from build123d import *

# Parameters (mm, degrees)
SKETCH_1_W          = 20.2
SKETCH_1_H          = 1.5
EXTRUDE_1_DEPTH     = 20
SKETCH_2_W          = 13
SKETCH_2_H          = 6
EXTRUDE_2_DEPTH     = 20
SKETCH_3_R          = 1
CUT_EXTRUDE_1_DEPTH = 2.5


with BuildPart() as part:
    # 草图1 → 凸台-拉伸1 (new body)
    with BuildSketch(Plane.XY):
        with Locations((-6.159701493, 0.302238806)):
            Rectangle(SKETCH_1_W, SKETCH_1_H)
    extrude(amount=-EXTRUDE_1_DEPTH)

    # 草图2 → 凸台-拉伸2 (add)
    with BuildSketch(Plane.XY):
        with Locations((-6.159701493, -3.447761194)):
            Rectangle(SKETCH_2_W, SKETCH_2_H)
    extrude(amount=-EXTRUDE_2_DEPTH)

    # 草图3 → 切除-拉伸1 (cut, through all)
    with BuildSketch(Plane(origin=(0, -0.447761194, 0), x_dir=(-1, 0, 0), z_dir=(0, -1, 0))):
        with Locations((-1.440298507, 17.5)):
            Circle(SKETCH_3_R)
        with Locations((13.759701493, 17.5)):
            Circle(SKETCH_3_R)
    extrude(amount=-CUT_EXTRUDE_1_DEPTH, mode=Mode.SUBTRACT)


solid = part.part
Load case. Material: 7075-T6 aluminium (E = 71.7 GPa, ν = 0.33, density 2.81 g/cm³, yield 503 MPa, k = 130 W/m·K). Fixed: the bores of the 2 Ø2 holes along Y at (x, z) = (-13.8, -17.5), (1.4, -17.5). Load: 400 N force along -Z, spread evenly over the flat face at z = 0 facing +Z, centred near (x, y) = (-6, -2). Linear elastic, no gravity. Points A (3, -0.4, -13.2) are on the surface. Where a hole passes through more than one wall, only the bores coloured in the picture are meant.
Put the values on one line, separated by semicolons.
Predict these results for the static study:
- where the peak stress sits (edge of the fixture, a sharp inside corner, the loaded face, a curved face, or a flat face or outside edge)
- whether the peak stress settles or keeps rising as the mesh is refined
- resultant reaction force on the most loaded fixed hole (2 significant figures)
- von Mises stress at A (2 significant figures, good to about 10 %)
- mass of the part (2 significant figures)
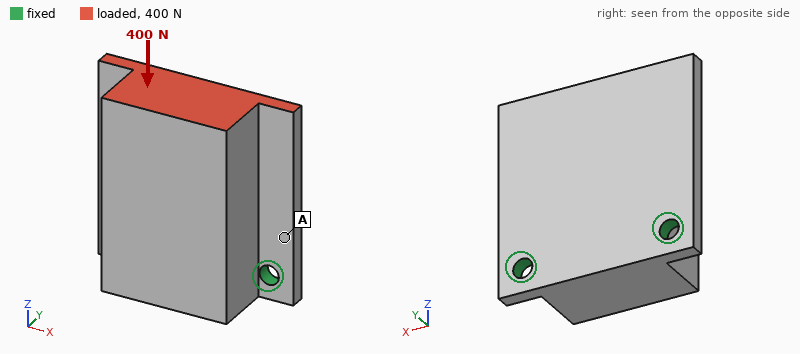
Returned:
edge of the fixture; keeps rising; 200 N; 22 MPa; 6.1 g
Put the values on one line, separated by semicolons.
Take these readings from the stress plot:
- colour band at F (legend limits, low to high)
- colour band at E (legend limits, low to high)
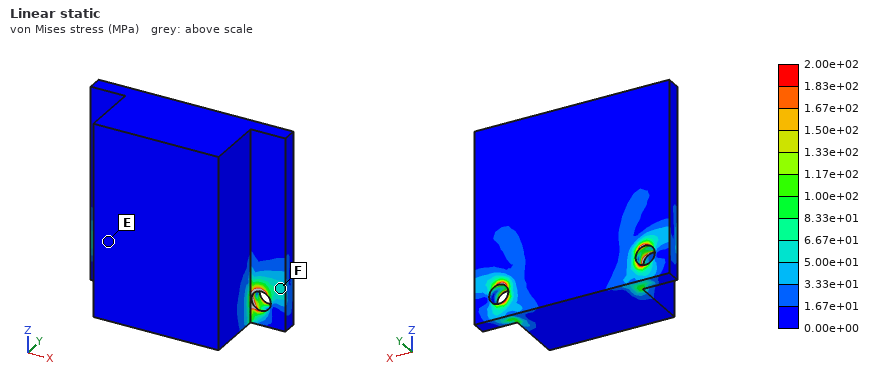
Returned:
5.00e+01 to 6.67e+01 MPa; 0.00e+00 to 1.67e+01 MPa
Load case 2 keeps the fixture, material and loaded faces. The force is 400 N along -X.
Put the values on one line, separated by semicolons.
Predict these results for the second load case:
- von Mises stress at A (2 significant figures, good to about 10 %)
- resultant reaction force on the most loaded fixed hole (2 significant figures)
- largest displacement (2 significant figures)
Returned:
34 MPa; 500 N; 14 µm
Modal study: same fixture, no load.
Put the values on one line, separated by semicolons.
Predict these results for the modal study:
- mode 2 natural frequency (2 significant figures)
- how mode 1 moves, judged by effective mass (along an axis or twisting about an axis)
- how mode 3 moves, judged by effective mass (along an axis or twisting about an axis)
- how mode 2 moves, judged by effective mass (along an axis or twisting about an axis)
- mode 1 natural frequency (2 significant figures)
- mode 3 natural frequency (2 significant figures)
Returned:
21 kHz; along Y; twisting about Z; along X; 3900 Hz; 25 kHz
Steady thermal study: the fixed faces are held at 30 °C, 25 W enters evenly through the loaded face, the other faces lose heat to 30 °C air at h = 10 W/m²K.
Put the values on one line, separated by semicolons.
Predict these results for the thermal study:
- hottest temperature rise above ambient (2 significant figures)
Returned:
48 K
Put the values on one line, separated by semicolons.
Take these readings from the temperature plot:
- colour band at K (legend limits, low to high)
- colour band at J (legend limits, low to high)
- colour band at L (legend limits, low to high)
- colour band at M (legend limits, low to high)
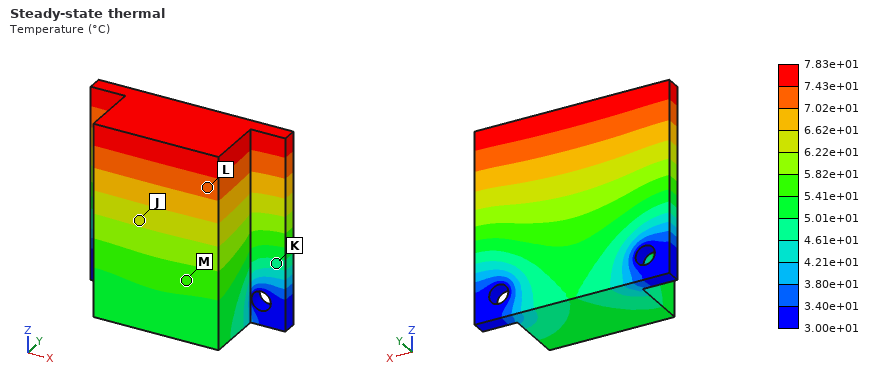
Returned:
4.61e+01 to 5.01e+01 °C; 6.22e+01 to 6.62e+01 °C; 7.02e+01 to 7.43e+01 °C; 5.41e+01 to 5.82e+01 °C
